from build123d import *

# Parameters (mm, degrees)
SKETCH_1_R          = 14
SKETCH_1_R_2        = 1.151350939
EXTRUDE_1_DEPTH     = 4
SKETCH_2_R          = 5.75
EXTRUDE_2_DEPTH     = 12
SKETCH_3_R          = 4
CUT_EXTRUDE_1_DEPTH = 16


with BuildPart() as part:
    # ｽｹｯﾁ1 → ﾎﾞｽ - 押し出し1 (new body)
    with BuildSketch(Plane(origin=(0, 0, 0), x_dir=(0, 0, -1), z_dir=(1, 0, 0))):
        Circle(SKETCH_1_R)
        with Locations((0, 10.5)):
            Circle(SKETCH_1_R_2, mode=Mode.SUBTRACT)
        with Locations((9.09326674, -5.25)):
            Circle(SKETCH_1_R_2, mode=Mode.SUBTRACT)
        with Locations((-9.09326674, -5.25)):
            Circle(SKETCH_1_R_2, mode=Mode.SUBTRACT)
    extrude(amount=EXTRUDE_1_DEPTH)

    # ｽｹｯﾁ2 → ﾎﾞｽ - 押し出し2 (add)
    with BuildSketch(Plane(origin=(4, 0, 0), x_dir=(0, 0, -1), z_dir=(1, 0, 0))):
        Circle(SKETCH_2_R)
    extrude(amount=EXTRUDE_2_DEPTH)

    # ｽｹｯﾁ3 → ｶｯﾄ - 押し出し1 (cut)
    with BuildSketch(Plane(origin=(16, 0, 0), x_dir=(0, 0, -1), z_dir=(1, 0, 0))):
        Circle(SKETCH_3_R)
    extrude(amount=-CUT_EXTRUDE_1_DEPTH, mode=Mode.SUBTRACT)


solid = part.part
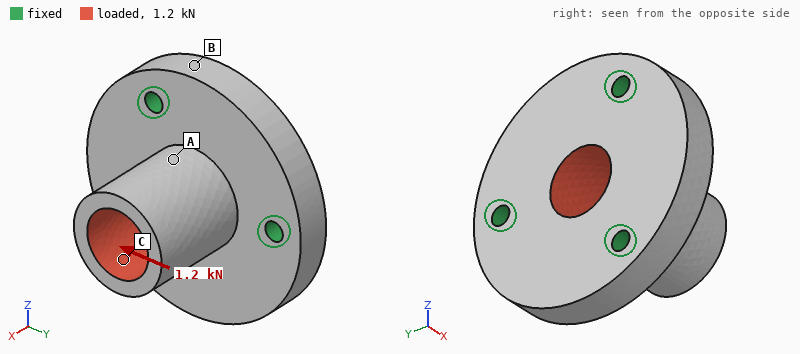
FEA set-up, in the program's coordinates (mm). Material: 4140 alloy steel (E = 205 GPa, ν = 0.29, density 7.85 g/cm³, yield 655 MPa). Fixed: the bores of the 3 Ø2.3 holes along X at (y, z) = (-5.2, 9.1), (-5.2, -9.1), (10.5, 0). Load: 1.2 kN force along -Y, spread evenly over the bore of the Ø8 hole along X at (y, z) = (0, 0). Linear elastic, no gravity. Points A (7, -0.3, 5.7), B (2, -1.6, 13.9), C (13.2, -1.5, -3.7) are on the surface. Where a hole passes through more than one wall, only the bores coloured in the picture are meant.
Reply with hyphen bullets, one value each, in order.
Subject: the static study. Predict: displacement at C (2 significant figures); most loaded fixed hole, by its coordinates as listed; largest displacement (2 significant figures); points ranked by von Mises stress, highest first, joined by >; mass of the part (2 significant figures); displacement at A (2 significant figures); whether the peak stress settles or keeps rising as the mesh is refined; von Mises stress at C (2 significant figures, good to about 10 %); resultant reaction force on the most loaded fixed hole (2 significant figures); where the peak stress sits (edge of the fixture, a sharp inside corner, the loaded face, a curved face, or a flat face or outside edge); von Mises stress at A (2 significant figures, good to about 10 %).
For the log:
- 7.1 µm
- (10.5, 0)
- 9.2 µm
- A > C > B
- 22 g
- 2.9 µm
- keeps rising
- 17 MPa
- 620 N
- edge of the fixture
- 29 MPa
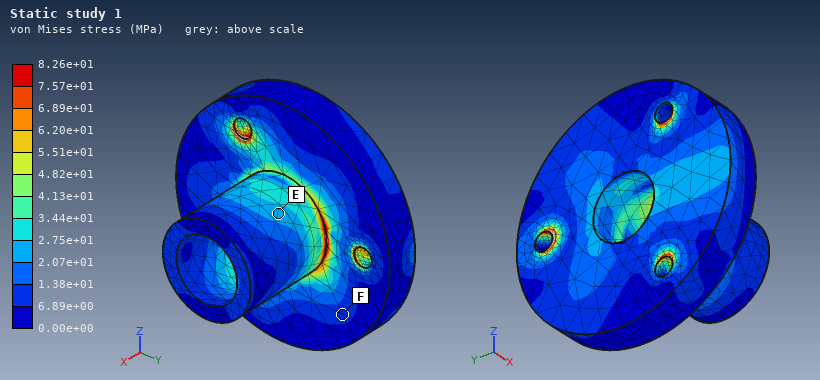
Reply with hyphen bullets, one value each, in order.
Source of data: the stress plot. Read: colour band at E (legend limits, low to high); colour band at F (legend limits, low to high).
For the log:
- 2.07e+01 to 2.75e+01 MPa
- 6.89e+00 to 1.38e+01 MPa
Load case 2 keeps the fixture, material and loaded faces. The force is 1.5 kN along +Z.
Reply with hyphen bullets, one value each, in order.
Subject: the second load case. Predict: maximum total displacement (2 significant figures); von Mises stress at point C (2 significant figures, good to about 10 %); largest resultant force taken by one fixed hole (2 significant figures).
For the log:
- 11 µm
- 18 MPa
- 710 N
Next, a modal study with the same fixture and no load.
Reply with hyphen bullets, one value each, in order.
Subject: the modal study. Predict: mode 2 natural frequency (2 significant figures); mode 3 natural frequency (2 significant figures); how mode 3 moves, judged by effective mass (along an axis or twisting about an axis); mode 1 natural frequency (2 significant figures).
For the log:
- 24 kHz
- 35 kHz
- along X
- 24 kHz
